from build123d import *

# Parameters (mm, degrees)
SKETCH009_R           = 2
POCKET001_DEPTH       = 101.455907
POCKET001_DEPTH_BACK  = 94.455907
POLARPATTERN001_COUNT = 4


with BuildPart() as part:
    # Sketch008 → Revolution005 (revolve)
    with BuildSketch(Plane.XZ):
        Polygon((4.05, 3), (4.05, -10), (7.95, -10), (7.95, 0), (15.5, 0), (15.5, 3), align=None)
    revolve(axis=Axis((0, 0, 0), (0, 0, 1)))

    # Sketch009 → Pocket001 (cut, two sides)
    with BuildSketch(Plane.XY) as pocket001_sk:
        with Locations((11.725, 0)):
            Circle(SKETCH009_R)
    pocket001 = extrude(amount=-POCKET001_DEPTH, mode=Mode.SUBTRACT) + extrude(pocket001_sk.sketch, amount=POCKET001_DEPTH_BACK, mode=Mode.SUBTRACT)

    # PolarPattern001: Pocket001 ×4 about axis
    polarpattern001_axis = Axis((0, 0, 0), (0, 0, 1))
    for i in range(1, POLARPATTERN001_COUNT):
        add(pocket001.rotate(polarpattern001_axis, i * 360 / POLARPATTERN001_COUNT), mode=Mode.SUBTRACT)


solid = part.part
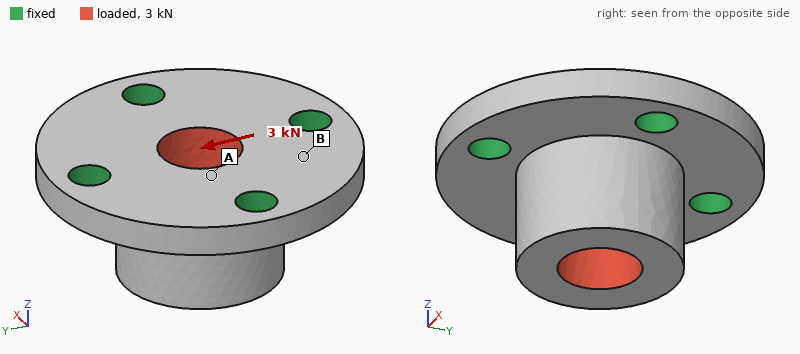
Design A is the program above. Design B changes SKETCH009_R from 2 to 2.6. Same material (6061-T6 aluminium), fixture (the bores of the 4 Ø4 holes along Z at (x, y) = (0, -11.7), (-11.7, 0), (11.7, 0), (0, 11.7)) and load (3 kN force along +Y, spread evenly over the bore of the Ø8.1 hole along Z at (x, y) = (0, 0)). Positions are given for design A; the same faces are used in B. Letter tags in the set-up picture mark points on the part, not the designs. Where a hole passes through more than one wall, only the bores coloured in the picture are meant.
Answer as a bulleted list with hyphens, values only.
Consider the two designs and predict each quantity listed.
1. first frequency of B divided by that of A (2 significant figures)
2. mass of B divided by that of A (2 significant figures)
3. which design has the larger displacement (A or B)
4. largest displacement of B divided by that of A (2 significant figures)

- 1.1
- 0.97
- A
- 0.85
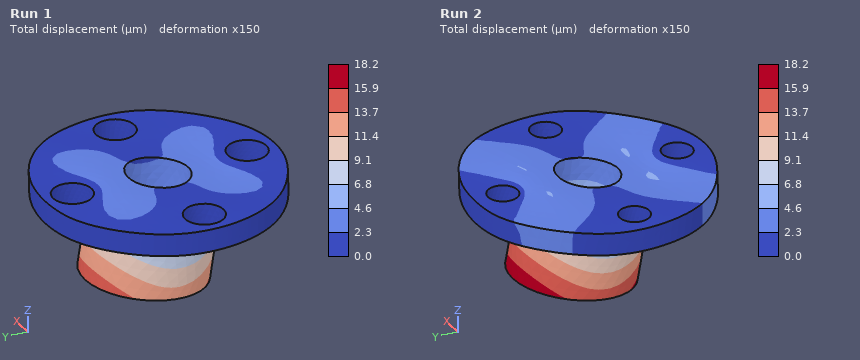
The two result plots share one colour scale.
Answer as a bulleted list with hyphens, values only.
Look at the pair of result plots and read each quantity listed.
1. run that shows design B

- Run 1
